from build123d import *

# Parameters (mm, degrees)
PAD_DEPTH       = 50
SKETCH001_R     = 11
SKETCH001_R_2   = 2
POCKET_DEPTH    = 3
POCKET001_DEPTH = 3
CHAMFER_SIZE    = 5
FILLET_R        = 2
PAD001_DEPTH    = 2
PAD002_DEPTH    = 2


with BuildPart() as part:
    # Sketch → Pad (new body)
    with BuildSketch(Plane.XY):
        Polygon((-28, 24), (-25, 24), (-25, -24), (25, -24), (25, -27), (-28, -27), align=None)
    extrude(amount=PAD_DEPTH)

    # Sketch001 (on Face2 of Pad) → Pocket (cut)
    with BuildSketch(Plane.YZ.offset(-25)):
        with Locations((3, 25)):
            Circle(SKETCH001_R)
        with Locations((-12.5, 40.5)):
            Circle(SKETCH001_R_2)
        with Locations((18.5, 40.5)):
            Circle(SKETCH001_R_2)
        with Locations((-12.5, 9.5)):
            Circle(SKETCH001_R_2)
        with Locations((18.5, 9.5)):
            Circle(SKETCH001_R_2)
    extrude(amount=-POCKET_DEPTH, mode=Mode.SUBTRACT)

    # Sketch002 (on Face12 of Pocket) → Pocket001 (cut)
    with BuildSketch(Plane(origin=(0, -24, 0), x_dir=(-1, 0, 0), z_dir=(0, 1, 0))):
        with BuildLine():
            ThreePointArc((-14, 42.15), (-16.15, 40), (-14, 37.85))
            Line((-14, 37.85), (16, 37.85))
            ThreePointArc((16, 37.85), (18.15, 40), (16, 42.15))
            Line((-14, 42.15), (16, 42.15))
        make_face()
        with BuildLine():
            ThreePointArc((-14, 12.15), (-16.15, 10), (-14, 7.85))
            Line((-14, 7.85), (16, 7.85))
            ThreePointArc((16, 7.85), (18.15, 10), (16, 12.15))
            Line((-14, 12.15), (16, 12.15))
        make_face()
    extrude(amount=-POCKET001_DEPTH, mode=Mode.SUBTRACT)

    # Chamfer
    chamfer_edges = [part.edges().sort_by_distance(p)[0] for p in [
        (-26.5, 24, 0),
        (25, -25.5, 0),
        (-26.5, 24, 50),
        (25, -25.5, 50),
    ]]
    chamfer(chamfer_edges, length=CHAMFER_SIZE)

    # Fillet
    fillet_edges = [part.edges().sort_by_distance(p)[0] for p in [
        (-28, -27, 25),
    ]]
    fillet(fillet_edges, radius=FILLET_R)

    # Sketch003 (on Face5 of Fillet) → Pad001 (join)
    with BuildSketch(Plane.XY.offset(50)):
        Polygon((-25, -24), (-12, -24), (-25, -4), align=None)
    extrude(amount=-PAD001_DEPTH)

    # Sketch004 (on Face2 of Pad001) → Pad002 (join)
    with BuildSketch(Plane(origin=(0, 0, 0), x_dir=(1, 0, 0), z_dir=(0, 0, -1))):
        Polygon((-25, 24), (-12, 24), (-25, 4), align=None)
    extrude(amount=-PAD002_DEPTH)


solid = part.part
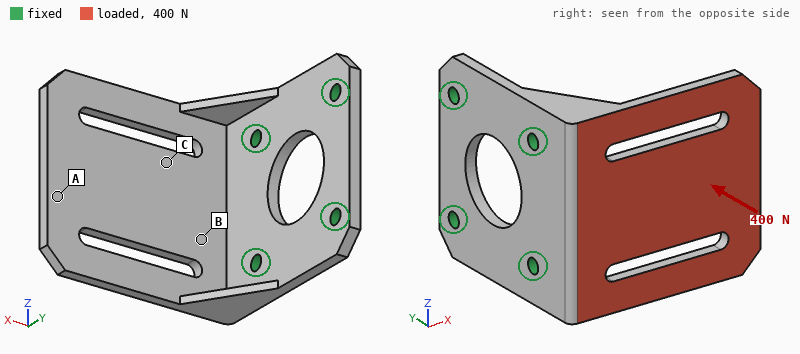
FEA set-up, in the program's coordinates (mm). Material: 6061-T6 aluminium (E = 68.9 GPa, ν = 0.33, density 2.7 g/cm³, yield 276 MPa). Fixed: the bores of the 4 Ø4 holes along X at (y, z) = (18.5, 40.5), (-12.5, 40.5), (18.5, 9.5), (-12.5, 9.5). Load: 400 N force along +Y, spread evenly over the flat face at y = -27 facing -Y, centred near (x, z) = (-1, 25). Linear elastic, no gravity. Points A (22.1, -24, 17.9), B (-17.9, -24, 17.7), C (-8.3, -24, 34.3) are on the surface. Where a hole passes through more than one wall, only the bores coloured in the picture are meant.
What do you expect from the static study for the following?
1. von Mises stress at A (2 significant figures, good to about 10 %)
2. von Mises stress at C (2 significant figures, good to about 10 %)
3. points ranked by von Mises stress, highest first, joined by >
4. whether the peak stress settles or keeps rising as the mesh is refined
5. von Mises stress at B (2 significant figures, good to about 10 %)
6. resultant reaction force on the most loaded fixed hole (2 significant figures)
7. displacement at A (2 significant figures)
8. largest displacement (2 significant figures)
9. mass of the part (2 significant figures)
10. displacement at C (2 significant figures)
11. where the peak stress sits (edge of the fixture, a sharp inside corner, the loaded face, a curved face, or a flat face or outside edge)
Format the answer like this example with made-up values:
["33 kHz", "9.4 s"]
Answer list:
["20 MPa", "45 MPa", "B > C > A", "keeps rising", "67 MPa", "210 N", "0.94 mm", "1.0 mm", "36 g", "0.25 mm", "edge of the fixture"]
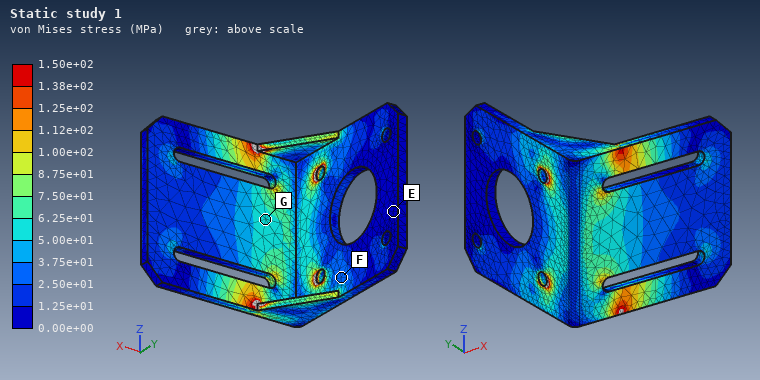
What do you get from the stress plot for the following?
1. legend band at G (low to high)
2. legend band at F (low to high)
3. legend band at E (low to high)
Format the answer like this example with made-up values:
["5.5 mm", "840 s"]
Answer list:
["5.00e+01 to 6.25e+01 MPa", "2.50e+01 to 3.75e+01 MPa", "0.00e+00 to 1.25e+01 MPa"]
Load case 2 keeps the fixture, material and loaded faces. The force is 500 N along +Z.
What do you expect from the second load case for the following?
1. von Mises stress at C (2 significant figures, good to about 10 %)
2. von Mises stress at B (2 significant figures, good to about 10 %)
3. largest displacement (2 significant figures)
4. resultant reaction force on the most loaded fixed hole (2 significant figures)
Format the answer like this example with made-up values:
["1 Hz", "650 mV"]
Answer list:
["10 MPa", "21 MPa", "0.14 mm", "490 N"]
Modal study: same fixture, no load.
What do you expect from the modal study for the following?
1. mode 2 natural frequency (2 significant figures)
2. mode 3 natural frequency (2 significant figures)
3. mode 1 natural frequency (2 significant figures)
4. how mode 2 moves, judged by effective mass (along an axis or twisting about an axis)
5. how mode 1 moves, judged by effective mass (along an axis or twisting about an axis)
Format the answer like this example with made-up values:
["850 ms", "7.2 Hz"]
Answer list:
["2100 Hz", "3200 Hz", "920 Hz", "along Z", "along Y"]
